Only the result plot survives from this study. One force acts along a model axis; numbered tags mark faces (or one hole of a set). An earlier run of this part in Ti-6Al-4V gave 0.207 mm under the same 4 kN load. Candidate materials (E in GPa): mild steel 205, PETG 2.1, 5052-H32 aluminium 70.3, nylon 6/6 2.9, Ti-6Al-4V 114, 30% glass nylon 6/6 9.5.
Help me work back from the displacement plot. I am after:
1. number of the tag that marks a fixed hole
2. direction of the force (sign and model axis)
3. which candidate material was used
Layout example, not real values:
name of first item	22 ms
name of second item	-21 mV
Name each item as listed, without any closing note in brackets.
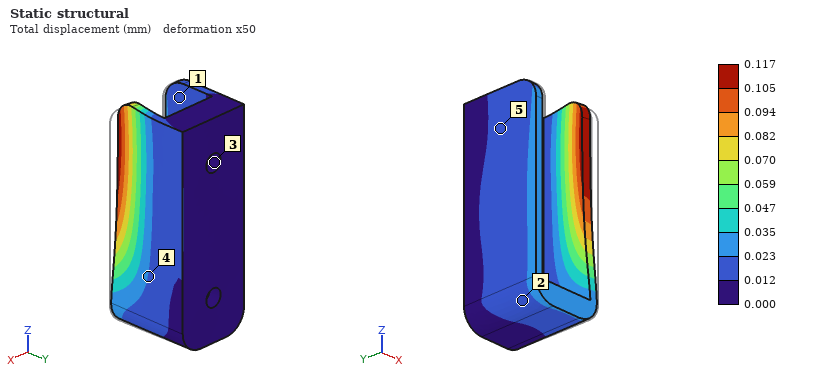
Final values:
number of the tag that marks a fixed hole	3
direction of the force	-X
which candidate material was used	mild steel
